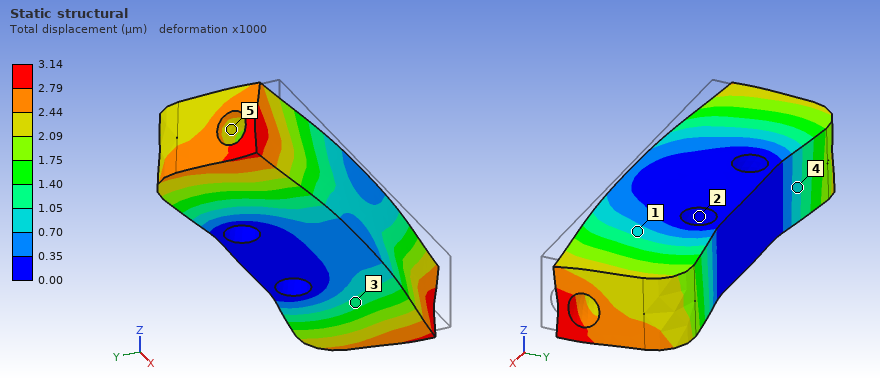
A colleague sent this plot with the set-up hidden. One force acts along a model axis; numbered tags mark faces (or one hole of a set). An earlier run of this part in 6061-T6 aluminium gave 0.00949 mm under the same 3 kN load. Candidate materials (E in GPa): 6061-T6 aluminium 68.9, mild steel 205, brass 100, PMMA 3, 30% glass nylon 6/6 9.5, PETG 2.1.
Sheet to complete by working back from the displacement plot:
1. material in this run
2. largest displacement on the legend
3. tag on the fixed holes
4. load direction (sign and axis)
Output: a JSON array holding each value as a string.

["mild steel", "3.14 µm", "2", "+Y"]
